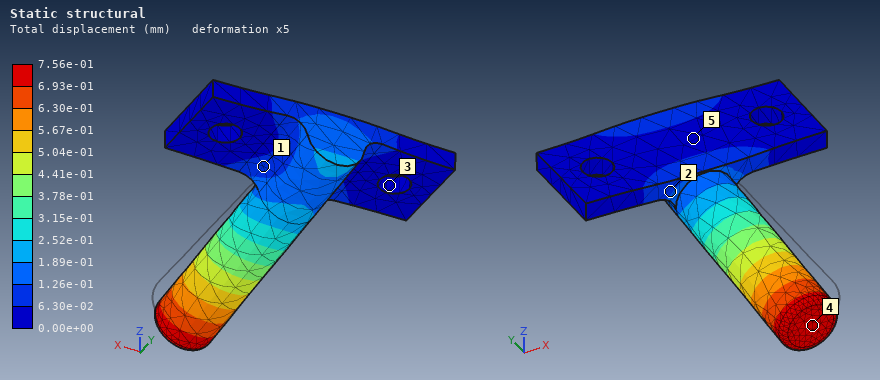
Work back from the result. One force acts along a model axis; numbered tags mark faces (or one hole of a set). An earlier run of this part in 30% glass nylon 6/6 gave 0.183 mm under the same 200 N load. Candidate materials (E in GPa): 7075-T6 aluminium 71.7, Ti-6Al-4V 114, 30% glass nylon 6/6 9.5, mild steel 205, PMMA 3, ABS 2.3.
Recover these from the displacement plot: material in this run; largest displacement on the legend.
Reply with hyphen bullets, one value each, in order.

- ABS
- 7.56e-01 mm
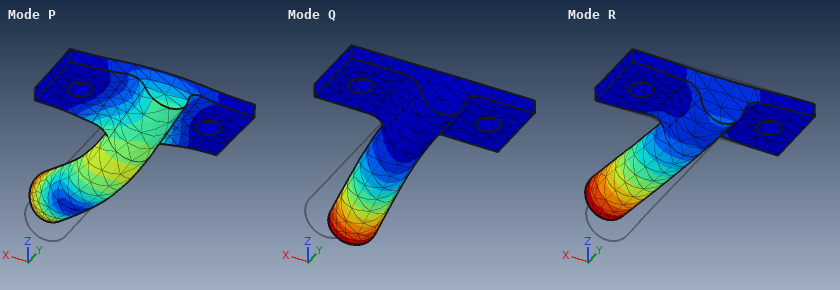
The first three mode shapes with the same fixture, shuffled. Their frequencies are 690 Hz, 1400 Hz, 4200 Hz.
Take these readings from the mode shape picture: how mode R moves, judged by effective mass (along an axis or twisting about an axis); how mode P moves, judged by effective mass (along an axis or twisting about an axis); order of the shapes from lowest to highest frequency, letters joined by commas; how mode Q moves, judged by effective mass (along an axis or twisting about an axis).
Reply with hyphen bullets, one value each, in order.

- along Z
- along Y
- R, Q, P
- along X
